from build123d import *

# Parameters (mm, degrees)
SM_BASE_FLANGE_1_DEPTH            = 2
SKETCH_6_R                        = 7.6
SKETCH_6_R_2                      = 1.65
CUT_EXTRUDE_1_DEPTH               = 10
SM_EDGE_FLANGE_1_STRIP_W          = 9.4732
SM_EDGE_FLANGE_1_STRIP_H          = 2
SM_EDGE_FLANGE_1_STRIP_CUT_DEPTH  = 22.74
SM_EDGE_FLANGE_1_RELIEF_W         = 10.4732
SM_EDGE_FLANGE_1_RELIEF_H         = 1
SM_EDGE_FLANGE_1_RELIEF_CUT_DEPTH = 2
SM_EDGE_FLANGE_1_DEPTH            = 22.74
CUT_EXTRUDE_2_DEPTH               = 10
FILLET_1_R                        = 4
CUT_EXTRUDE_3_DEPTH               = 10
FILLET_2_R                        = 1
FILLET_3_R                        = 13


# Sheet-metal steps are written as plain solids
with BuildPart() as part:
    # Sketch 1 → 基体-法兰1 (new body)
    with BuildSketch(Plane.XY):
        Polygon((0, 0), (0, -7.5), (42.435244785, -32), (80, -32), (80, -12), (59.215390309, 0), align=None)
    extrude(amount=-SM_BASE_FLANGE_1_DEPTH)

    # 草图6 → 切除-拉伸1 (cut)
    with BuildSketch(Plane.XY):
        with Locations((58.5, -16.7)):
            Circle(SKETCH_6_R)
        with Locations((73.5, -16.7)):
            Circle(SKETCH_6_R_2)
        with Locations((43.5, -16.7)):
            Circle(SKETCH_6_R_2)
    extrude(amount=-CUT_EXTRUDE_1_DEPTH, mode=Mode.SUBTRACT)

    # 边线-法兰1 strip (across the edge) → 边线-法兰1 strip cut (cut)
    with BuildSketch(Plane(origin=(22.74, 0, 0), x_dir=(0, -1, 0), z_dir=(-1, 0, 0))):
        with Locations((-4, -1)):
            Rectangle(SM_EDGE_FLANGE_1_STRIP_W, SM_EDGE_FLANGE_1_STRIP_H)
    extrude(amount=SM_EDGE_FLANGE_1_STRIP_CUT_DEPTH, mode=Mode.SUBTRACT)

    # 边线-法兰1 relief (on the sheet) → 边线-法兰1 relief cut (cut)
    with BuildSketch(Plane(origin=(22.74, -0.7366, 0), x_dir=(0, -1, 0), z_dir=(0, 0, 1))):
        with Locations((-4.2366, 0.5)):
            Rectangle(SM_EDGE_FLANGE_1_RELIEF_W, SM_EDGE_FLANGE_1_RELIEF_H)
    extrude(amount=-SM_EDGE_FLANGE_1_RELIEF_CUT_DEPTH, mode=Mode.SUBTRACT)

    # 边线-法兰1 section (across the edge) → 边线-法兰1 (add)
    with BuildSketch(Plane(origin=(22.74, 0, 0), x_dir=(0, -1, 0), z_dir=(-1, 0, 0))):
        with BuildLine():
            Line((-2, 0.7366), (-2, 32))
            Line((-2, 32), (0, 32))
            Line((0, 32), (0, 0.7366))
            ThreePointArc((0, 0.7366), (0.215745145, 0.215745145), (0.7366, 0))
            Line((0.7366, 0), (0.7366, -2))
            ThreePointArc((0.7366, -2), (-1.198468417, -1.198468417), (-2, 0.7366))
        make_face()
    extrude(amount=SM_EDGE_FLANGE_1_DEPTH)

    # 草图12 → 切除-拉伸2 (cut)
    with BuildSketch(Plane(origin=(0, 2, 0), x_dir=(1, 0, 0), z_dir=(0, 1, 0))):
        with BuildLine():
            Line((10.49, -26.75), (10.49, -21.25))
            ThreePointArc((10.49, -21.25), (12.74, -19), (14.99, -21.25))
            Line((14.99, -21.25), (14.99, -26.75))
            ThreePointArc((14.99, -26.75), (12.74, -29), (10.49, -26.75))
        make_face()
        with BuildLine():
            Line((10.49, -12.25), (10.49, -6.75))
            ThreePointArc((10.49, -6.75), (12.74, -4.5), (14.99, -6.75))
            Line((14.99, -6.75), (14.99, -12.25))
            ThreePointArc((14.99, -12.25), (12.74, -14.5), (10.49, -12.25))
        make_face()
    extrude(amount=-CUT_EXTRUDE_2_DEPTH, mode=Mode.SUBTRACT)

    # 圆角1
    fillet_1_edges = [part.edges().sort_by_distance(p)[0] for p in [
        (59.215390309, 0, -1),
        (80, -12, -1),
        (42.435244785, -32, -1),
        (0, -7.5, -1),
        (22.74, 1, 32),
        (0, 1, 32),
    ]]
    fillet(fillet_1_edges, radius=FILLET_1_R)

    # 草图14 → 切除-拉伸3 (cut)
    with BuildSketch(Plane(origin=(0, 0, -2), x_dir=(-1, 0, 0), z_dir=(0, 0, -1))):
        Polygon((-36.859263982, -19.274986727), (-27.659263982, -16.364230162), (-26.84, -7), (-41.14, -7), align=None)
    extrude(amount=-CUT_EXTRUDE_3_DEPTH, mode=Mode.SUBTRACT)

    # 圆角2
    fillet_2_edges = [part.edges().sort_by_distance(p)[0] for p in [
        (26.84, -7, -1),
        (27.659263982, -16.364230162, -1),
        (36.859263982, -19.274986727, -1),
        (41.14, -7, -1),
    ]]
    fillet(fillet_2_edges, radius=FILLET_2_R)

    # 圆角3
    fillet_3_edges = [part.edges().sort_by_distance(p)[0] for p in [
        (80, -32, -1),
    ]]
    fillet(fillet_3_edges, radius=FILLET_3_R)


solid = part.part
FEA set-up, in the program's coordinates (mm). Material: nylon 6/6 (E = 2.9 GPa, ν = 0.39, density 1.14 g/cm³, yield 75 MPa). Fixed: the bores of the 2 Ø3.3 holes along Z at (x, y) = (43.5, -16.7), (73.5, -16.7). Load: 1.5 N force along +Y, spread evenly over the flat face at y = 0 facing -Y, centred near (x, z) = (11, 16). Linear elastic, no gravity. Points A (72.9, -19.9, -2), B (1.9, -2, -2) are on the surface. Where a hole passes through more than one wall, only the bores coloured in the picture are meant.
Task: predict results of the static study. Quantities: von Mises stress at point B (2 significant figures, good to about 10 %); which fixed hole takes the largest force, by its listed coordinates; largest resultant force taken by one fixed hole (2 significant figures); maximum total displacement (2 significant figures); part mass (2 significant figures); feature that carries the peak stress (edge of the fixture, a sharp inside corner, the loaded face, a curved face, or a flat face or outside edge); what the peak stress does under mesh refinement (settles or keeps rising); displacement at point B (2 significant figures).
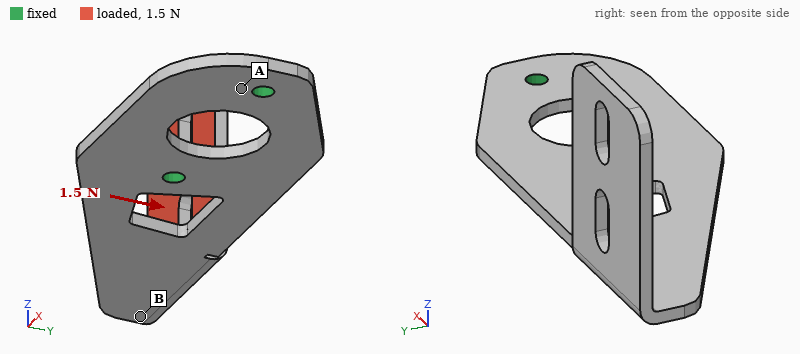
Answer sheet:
1.1 MPa
(43.5, -16.7)
2.8 N
0.94 mm
5.1 g
a sharp inside corner
keeps rising
0.26 mm
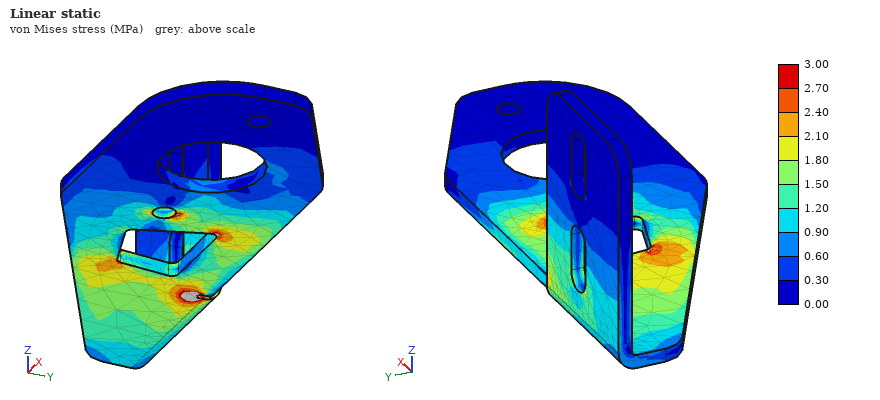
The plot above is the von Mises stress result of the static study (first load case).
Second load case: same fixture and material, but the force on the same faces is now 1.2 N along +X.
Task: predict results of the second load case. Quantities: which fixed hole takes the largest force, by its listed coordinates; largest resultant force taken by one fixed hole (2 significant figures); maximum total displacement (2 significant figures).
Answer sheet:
(43.5, -16.7)
0.93 N
0.93 mm
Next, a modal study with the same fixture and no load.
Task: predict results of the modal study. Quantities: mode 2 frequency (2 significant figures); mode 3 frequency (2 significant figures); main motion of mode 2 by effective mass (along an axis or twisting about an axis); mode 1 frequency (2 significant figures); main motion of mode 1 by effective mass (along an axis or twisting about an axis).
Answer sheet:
230 Hz
500 Hz
along Y
120 Hz
along Z
